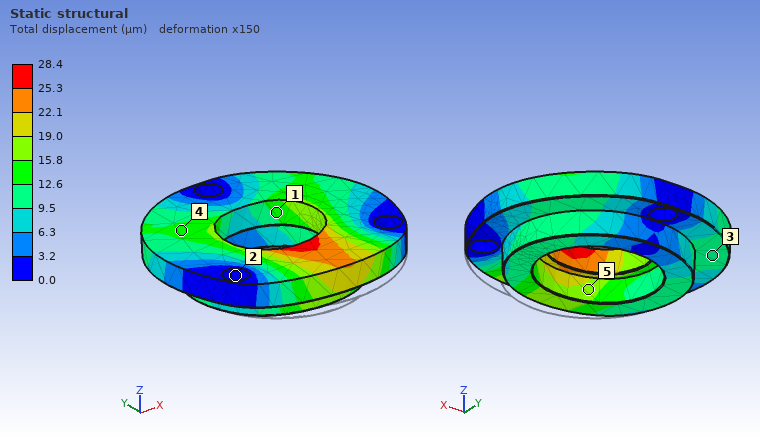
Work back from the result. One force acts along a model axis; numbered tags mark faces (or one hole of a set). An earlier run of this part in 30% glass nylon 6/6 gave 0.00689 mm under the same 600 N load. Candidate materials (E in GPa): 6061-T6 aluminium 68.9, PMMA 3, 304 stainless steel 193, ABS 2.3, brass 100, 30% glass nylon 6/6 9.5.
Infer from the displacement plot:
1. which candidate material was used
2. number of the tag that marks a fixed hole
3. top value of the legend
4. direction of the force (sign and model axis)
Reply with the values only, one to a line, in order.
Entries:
ABS
2
28.4 µm
+Y
